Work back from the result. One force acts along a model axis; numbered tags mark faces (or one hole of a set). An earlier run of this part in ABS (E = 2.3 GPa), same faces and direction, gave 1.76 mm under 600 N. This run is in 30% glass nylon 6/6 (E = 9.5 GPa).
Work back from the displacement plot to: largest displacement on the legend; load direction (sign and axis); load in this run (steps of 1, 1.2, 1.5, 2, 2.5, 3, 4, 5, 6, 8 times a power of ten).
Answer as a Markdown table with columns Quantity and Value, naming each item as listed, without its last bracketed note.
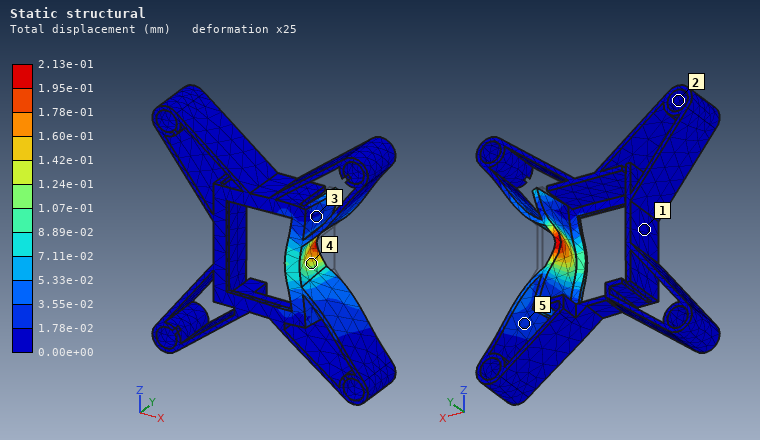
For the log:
| Quantity | Value |
|---|---|
| largest displacement on the legend | 2.13e-01 mm |
| load direction | -X |
| load in this run | 300 N |
